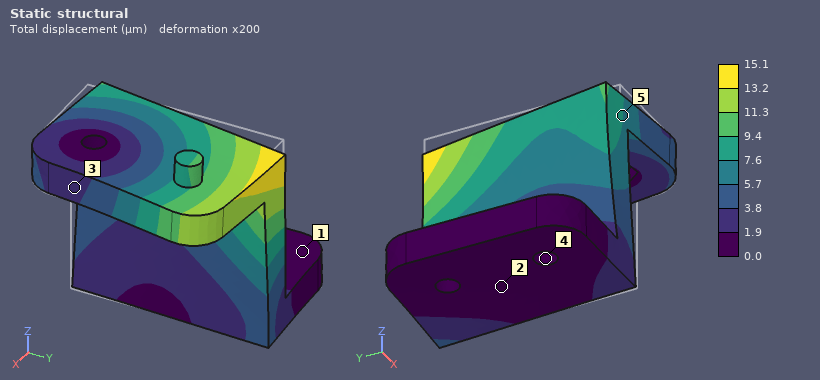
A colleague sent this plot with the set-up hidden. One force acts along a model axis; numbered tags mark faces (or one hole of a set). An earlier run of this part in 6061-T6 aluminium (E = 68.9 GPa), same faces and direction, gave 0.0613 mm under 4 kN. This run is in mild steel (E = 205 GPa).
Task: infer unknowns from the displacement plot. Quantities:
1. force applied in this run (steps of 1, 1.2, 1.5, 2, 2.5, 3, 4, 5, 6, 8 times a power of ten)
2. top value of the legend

3 kN
15.1 µm
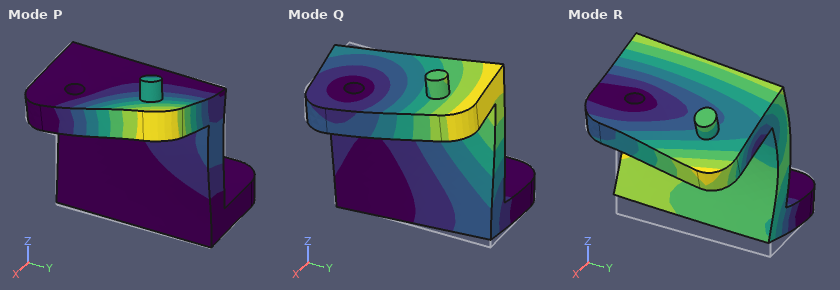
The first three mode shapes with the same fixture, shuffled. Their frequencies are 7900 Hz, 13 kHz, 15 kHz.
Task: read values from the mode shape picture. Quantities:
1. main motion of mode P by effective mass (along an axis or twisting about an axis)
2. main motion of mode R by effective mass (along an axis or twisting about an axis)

along Z
along Z
